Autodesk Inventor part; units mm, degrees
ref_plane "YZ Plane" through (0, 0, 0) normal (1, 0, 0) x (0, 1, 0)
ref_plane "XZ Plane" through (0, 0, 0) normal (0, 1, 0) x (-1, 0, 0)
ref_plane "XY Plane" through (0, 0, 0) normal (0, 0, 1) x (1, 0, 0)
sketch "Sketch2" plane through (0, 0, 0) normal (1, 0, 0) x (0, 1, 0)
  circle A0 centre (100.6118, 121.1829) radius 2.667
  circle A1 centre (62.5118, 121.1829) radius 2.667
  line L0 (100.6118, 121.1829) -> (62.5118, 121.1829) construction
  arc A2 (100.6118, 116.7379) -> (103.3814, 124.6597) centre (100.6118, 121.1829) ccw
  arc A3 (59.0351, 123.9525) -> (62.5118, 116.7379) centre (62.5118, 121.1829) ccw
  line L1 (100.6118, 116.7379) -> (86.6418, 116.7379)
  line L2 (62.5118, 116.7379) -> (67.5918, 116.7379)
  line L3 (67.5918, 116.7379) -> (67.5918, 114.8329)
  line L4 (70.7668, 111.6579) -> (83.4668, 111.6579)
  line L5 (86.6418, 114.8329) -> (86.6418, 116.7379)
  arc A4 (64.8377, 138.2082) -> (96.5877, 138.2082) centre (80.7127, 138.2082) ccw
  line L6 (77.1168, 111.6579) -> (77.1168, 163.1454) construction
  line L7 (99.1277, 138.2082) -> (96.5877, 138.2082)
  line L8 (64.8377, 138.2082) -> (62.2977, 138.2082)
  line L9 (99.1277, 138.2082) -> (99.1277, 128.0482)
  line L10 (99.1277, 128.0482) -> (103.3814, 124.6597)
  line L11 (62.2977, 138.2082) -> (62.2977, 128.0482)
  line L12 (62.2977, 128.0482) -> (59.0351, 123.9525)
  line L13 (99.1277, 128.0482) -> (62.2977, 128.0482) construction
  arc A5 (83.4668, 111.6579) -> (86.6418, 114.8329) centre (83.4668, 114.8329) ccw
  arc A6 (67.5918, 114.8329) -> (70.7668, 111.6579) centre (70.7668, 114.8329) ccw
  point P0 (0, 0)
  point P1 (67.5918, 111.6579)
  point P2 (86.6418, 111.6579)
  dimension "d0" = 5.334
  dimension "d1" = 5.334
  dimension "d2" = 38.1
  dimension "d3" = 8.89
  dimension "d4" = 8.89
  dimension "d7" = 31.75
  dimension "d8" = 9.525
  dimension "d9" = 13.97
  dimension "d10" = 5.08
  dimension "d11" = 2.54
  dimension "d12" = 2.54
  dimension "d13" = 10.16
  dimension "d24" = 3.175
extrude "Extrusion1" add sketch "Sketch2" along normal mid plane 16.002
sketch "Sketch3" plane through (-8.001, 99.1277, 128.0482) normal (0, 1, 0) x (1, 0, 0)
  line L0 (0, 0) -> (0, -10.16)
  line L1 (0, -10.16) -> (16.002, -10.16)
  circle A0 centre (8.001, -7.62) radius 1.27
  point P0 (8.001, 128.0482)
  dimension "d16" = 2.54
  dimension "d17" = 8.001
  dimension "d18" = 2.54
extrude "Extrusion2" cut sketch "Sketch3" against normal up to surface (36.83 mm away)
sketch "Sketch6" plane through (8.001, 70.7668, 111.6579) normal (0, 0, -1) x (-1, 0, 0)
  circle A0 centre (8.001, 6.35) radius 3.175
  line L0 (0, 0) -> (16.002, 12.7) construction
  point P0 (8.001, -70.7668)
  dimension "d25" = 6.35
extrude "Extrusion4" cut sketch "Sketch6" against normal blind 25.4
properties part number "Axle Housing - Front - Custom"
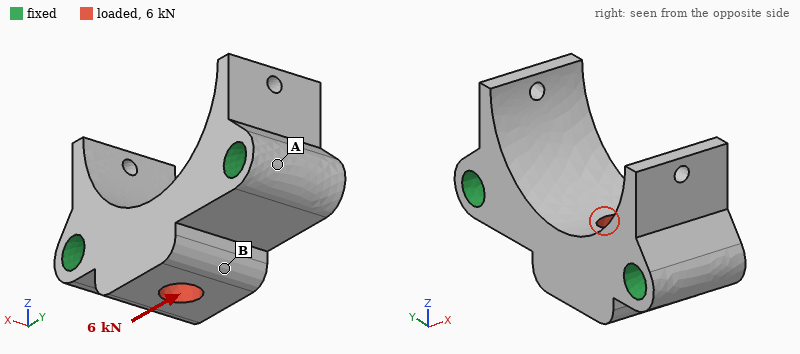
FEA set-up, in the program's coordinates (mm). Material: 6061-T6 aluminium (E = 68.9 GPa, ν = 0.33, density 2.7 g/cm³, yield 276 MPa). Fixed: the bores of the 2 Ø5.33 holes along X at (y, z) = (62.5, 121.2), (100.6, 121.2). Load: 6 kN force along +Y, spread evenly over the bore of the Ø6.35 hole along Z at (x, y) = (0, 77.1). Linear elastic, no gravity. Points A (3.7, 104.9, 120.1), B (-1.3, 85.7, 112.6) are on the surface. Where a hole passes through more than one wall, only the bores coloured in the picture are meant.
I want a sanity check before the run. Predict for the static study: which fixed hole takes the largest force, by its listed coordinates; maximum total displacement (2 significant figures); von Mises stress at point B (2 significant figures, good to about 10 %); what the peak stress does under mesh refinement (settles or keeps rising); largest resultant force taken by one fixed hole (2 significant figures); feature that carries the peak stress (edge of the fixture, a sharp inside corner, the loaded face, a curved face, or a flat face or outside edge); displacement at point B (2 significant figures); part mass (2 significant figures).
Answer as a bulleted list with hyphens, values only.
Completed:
- (62.5, 121.2)
- 9.5 µm
- 20 MPa
- keeps rising
- 3.7 kN
- edge of the fixture
- 7.8 µm
- 22 g
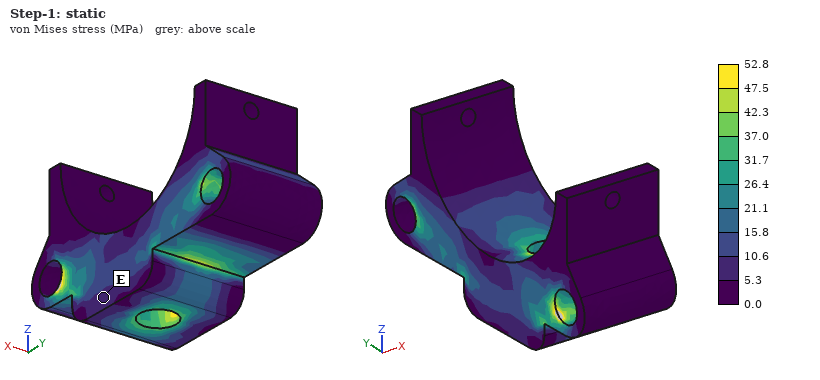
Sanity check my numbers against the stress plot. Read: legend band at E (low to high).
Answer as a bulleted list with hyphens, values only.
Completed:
- 5.3 to 10.6 MPa
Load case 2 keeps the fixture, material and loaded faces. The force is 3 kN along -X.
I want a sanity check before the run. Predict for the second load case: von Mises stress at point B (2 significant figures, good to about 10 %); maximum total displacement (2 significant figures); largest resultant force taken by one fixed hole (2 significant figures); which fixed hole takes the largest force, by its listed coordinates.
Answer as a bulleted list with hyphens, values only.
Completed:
- 7.6 MPa
- 16 µm
- 2.0 kN
- (62.5, 121.2)
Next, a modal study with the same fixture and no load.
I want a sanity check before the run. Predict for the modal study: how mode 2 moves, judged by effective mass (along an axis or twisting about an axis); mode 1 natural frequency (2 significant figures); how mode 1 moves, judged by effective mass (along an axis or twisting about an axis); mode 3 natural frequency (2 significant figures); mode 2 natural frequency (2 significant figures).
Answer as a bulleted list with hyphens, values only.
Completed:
- along X
- 24 kHz
- along Z
- 32 kHz
- 28 kHz
